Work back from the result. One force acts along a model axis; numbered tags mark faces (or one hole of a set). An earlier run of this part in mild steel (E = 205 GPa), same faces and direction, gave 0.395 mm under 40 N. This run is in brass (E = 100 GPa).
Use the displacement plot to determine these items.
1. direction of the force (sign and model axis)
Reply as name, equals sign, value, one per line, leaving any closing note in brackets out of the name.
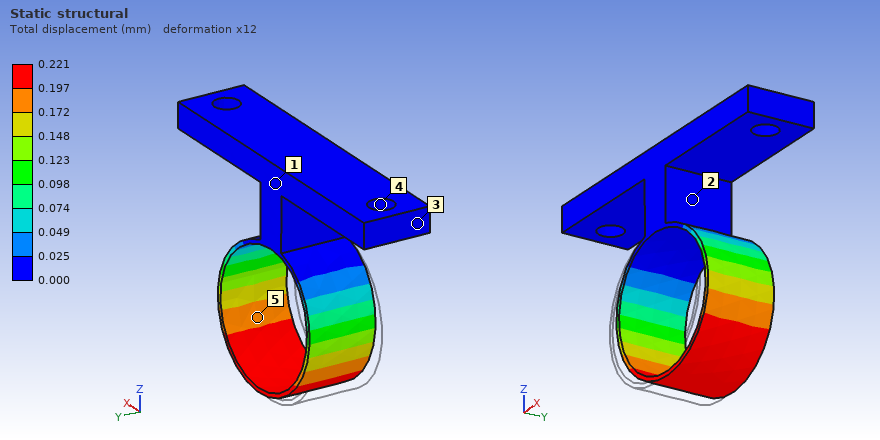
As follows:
direction of the force = +X
